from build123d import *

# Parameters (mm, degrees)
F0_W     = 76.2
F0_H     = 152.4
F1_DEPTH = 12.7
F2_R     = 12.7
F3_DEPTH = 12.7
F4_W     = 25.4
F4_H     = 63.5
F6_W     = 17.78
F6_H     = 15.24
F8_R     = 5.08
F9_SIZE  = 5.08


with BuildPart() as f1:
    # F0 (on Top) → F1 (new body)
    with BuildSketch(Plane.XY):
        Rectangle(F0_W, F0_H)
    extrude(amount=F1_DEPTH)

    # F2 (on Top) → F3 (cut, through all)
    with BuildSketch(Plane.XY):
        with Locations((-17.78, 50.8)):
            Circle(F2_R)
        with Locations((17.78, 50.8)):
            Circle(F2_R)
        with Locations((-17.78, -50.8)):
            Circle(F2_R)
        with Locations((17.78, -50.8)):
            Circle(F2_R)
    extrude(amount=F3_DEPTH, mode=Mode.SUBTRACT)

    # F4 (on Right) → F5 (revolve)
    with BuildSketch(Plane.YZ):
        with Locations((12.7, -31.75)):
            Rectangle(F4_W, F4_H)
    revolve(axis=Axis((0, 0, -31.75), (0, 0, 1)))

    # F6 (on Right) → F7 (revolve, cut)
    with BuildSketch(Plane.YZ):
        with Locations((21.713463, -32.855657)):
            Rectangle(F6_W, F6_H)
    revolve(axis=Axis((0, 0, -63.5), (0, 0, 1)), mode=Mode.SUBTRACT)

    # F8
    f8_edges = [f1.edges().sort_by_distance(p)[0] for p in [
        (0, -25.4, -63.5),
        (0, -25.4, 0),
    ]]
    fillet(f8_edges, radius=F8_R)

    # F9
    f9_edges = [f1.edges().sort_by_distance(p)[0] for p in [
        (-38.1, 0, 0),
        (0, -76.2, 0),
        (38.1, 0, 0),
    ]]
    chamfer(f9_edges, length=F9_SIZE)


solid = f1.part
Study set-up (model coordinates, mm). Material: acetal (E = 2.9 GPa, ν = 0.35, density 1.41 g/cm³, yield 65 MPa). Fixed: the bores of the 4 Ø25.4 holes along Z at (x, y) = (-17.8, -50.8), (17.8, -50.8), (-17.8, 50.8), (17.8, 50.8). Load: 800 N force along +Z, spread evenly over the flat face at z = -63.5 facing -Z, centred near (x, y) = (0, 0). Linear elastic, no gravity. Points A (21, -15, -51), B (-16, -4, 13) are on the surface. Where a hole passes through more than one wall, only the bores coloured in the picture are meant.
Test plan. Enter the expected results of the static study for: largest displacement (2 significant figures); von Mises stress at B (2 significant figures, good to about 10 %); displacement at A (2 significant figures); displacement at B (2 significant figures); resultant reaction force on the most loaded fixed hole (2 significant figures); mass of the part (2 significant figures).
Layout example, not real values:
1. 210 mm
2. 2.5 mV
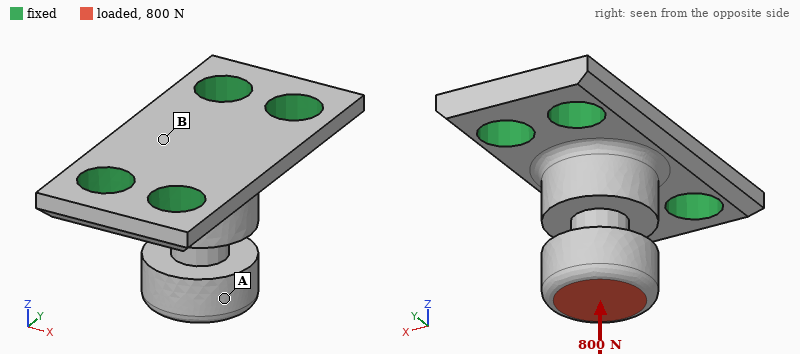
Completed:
1. 45 µm
2. 0.70 MPa
3. 43 µm
4. 26 µm
5. 220 N
6. 310 g
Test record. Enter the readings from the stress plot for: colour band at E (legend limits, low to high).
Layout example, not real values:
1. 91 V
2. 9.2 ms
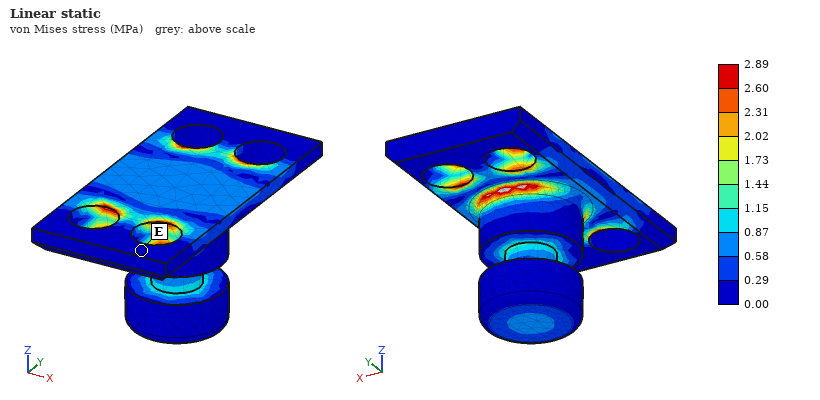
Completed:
1. 0.00 to 0.29 MPa
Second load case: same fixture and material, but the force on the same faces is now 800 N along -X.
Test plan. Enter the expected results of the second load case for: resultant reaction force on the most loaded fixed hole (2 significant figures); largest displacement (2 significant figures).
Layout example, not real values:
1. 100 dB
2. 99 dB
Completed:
1. 690 N
2. 0.80 mm
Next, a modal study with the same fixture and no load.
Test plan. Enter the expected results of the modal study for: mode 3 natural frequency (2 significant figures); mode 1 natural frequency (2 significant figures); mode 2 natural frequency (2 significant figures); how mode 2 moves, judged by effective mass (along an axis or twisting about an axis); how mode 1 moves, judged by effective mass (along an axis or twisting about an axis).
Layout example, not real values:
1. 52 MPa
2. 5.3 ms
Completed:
1. 1500 Hz
2. 760 Hz
3. 970 Hz
4. along Y
5. along X
